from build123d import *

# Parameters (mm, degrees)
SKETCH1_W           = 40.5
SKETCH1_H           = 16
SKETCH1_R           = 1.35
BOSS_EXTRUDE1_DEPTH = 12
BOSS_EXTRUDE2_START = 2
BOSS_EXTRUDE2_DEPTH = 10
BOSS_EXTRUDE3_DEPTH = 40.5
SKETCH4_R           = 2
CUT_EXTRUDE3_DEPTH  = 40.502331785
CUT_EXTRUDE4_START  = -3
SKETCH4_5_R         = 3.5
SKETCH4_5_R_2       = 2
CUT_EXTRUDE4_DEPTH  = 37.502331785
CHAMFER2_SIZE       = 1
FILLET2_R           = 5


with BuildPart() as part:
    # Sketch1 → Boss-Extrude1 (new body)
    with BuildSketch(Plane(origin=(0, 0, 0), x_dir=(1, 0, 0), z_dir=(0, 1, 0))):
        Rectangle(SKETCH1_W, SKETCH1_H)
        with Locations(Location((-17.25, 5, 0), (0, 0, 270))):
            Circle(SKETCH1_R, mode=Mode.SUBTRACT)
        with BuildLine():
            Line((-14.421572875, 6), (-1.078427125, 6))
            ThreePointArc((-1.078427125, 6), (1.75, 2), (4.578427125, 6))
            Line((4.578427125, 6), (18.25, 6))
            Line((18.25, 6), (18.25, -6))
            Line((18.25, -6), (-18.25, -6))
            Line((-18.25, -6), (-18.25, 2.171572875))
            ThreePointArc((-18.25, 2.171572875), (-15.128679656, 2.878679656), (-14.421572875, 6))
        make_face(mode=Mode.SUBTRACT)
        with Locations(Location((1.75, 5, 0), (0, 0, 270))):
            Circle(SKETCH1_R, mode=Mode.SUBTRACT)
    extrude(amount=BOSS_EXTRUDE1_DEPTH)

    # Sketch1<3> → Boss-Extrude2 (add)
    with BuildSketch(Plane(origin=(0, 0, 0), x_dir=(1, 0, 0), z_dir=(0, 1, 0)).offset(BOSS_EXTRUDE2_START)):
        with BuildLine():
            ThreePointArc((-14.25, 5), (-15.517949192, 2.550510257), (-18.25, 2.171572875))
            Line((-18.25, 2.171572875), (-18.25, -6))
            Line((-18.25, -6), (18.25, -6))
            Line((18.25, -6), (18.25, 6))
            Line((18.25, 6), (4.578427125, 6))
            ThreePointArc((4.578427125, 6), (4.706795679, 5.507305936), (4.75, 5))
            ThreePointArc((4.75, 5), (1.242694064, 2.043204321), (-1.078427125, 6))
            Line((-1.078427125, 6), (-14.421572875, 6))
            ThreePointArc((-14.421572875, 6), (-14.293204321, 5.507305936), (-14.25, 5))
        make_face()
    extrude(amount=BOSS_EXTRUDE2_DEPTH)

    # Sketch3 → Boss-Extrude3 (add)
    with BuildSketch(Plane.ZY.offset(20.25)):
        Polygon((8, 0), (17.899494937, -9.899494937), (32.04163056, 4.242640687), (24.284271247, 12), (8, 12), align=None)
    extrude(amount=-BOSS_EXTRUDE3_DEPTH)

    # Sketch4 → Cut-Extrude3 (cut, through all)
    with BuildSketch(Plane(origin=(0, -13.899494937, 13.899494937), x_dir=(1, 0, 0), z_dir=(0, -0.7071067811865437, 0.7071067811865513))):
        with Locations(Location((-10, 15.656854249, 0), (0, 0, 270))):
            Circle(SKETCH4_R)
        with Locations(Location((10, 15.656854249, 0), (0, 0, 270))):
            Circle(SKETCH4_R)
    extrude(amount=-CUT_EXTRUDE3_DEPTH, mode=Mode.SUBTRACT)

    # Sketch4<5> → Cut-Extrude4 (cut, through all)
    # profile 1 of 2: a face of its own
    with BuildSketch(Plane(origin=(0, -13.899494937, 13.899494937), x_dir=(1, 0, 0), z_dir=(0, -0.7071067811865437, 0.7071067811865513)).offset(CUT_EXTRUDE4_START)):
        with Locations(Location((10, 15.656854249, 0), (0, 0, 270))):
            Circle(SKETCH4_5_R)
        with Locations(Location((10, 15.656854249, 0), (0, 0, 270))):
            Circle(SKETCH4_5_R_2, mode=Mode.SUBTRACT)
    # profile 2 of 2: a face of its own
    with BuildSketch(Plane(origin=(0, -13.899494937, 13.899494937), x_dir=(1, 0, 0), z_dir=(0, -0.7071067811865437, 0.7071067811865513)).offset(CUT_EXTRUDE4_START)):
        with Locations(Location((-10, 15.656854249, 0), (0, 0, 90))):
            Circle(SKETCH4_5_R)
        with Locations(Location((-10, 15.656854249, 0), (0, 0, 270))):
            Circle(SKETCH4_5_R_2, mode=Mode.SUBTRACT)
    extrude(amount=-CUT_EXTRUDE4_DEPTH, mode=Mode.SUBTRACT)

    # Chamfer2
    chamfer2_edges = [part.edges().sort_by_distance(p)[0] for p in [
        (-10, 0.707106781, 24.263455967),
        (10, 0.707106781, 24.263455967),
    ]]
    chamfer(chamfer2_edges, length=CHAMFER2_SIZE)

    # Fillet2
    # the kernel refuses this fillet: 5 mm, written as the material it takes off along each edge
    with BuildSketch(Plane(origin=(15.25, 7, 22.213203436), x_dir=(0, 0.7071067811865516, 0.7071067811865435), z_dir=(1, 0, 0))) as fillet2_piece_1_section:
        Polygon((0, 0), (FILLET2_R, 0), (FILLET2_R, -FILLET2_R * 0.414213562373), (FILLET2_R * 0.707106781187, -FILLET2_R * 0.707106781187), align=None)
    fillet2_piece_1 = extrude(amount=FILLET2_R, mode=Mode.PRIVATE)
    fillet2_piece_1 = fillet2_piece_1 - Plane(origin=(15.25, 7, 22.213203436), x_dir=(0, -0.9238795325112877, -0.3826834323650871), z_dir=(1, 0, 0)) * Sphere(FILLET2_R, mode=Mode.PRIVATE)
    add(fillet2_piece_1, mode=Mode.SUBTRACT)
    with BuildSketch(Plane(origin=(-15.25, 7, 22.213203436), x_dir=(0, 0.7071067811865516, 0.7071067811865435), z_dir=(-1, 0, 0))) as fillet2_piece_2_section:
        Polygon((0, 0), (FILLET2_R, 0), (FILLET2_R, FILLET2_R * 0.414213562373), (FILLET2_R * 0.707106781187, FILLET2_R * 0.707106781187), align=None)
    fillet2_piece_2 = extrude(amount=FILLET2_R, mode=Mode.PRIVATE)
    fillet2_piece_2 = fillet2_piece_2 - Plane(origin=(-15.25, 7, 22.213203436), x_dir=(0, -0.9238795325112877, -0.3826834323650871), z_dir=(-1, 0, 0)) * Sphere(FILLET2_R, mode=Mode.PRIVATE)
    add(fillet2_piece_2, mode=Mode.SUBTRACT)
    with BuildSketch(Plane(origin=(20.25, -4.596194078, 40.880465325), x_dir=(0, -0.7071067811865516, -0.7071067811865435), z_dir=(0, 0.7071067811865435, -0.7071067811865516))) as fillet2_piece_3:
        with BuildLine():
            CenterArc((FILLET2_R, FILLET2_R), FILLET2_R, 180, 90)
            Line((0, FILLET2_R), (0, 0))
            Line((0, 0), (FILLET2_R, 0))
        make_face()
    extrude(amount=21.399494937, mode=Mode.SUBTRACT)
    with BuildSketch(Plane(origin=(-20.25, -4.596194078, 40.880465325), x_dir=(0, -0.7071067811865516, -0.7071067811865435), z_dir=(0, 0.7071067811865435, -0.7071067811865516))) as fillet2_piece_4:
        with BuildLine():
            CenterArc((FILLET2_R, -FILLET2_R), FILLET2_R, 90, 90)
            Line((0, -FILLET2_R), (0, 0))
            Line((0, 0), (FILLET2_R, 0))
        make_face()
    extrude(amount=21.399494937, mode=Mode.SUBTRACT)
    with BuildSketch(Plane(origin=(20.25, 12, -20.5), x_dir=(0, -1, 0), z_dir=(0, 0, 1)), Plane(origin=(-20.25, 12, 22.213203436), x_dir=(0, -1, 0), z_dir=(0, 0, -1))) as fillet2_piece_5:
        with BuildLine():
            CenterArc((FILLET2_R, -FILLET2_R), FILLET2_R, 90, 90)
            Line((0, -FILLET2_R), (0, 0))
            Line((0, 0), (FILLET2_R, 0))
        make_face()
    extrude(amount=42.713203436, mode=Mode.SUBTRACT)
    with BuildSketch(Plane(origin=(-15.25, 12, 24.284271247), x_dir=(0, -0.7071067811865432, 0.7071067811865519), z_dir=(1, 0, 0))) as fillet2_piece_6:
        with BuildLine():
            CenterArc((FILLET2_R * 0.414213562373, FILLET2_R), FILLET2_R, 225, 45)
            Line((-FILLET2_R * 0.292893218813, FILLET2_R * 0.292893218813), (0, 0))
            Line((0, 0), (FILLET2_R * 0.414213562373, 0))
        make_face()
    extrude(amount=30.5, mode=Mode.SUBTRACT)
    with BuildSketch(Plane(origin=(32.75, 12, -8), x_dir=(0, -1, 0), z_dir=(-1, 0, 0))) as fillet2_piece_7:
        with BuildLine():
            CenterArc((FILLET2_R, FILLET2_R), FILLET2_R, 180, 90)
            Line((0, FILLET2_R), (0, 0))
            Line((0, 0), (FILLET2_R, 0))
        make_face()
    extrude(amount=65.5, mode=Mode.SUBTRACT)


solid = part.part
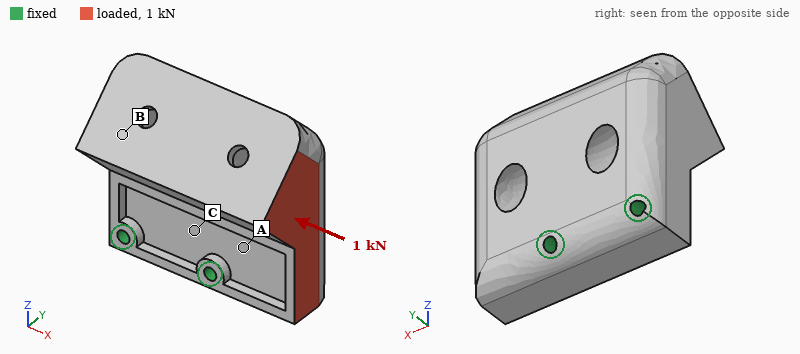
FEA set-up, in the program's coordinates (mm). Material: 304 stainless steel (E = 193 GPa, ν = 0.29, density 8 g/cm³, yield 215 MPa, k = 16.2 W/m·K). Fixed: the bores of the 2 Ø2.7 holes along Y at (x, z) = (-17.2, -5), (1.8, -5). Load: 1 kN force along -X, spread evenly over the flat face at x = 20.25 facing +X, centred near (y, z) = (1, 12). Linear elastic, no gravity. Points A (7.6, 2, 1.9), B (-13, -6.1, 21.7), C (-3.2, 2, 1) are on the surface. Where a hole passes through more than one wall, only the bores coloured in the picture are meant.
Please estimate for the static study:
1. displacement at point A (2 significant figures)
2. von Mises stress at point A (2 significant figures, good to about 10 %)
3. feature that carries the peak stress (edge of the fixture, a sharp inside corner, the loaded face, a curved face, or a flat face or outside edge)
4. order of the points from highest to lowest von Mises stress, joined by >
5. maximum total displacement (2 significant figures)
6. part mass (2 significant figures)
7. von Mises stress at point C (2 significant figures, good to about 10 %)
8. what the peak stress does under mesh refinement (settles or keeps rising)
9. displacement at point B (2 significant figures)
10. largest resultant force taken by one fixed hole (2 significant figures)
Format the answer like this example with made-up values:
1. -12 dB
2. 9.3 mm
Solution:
1. 1.3 µm
2. 7.7 MPa
3. edge of the fixture
4. C > A > B
5. 4.3 µm
6. 150 g
7. 13 MPa
8. keeps rising
9. 3.0 µm
10. 990 N
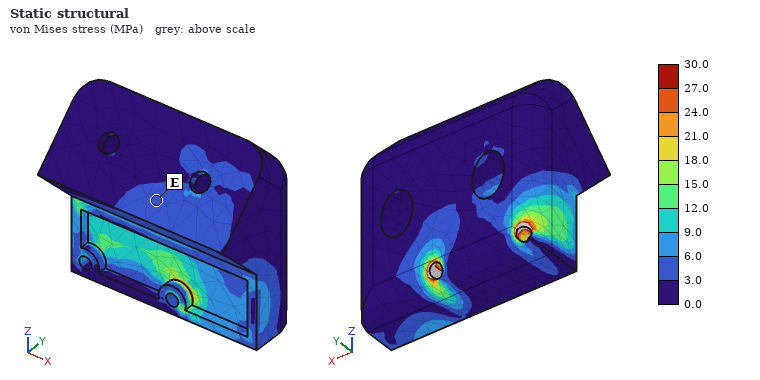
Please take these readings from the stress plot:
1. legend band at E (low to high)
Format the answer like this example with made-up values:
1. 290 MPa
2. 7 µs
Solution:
1. 3.0 to 6.0 MPa
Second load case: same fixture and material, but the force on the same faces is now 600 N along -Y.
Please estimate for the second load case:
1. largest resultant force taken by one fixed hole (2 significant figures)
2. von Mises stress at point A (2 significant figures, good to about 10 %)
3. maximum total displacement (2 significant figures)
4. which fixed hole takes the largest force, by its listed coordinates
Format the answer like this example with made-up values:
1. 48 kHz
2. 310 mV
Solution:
1. 880 N
2. 14 MPa
3. 14 µm
4. (1.8, -5)
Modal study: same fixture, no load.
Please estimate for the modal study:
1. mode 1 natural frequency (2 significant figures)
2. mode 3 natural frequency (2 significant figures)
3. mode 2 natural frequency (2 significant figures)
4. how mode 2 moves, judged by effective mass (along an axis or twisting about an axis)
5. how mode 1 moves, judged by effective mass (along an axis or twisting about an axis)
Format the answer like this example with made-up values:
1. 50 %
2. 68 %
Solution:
1. 4000 Hz
2. 9400 Hz
3. 7800 Hz
4. along X
5. along Y
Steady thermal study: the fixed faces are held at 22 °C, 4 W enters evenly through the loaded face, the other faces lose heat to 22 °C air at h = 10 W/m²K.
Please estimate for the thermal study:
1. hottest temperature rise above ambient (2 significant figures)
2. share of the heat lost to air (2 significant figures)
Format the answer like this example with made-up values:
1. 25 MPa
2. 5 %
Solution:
1. 22 K
2. 14 %
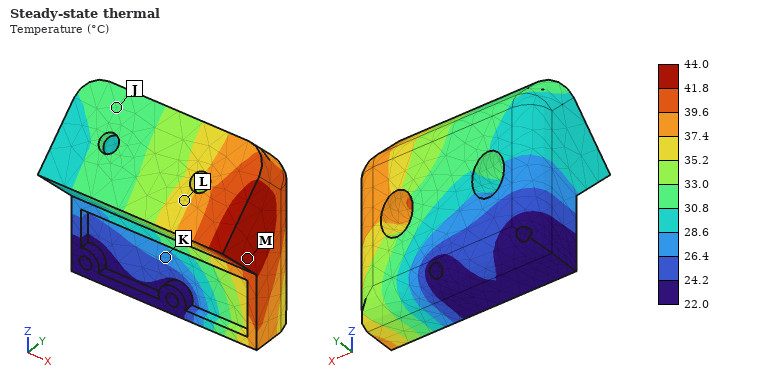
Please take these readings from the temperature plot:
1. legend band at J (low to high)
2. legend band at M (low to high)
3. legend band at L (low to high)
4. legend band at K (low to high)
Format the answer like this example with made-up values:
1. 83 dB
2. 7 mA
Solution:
1. 30.8 to 33.0 °C
2. 41.8 to 44.0 °C
3. 35.2 to 37.4 °C
4. 26.4 to 28.6 °C
